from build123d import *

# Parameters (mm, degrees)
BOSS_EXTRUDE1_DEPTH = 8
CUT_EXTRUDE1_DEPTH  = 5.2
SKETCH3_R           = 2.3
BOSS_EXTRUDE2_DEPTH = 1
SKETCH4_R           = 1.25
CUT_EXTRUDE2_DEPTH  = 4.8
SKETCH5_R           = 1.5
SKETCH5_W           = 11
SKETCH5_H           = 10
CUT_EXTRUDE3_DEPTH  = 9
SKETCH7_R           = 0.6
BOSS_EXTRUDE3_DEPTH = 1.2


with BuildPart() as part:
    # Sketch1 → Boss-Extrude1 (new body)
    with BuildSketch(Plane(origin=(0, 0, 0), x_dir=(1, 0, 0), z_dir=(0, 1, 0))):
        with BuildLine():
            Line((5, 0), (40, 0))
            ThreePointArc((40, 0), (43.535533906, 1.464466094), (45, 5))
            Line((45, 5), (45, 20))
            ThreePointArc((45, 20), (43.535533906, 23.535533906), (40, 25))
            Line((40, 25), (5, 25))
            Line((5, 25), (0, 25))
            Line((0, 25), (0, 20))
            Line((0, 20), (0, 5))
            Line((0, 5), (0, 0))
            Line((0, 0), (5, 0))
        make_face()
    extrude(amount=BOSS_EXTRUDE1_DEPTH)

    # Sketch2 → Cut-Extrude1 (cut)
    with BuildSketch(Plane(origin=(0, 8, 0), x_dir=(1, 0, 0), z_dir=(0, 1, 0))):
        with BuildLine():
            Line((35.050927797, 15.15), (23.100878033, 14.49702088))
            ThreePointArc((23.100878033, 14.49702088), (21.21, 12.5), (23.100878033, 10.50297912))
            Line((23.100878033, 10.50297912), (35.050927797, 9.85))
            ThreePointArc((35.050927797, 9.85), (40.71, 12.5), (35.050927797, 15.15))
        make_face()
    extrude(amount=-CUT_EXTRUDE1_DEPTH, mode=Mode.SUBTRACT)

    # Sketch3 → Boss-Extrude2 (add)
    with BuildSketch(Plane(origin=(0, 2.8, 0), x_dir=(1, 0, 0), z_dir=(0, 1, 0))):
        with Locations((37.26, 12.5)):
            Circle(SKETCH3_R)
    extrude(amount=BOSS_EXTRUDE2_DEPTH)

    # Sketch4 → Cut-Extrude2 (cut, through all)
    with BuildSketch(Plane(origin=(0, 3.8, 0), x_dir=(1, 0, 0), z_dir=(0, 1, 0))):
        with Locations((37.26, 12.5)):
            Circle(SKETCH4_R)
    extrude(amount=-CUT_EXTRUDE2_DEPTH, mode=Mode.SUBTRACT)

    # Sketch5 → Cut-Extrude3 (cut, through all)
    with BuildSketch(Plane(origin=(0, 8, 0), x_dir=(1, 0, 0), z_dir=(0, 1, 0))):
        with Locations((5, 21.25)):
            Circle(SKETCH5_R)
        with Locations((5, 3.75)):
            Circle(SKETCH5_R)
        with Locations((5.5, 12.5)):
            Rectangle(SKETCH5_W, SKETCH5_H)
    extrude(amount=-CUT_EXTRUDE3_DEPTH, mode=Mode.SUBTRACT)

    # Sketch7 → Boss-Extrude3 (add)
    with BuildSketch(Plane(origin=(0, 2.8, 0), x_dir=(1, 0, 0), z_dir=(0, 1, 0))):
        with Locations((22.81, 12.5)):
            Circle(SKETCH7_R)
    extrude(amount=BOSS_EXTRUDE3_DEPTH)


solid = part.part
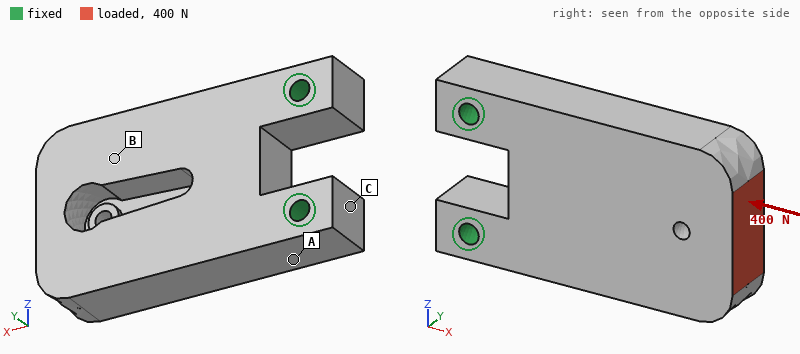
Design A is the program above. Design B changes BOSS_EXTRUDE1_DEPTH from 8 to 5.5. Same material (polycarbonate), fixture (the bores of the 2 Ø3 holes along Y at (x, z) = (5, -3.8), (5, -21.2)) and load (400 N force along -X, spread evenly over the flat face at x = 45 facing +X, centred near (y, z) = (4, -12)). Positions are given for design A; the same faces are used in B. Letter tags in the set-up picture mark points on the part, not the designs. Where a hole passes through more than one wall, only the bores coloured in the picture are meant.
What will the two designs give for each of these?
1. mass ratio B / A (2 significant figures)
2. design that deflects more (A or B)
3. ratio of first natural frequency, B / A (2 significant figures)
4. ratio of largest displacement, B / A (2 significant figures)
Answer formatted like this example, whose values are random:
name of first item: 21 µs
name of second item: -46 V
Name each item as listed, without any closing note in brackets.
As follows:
mass ratio B / A: 0.70
design that deflects more: B
ratio of first natural frequency, B / A: 0.70
ratio of largest displacement, B / A: 1.4
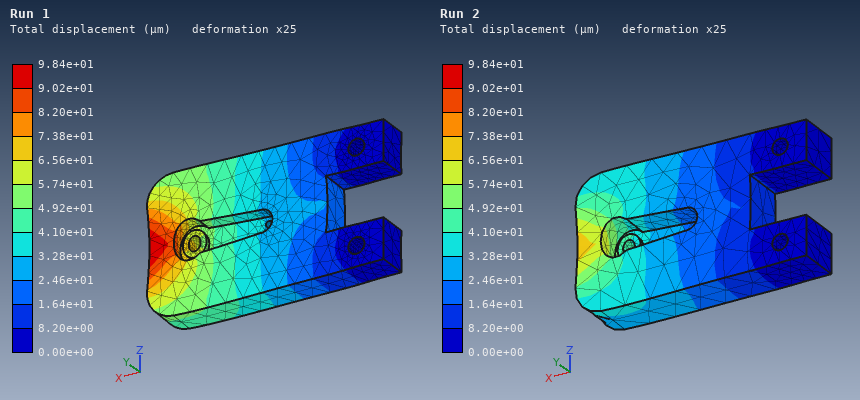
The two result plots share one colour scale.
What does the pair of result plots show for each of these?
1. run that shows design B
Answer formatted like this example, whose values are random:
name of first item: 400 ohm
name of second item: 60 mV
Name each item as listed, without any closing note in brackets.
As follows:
run that shows design B: Run 1
